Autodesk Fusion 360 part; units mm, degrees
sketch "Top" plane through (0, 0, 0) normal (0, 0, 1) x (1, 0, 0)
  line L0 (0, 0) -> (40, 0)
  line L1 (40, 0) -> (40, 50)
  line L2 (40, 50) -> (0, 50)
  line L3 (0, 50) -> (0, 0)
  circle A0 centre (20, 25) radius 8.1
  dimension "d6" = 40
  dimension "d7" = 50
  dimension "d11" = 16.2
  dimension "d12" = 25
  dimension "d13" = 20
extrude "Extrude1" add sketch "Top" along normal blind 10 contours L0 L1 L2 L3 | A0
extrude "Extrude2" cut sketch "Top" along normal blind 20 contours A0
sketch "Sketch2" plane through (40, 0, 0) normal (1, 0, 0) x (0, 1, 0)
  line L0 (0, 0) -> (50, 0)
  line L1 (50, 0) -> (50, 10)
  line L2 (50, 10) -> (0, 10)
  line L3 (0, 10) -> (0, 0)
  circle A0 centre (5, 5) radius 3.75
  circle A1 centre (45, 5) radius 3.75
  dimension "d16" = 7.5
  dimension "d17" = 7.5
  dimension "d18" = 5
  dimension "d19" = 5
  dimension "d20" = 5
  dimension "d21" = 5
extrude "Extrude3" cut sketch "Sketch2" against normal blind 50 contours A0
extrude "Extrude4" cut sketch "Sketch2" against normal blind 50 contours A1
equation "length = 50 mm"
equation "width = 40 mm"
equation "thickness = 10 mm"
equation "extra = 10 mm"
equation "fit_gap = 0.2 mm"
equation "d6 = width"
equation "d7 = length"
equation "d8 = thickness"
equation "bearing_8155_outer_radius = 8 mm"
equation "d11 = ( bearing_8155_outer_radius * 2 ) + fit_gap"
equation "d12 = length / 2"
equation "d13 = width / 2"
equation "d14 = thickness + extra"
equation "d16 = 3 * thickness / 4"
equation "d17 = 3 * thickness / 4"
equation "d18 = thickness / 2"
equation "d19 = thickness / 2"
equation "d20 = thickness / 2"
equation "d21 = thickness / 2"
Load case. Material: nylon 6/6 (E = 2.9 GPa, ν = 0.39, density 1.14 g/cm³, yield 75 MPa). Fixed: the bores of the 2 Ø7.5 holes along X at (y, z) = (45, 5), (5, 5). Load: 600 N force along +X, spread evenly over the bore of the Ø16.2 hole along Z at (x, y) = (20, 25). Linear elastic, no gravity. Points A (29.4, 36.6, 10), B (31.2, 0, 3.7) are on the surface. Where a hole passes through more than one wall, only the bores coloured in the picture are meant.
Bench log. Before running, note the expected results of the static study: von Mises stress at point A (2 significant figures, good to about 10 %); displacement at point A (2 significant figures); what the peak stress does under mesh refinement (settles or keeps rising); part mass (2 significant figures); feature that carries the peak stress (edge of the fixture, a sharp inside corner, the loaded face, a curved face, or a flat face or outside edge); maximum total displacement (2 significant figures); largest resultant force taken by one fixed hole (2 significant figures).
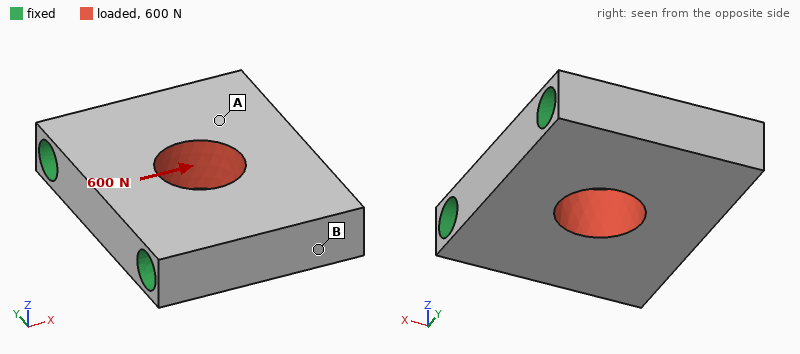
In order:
1.3 MPa
4.2 µm
keeps rising
16 g
edge of the fixture
13 µm
300 N
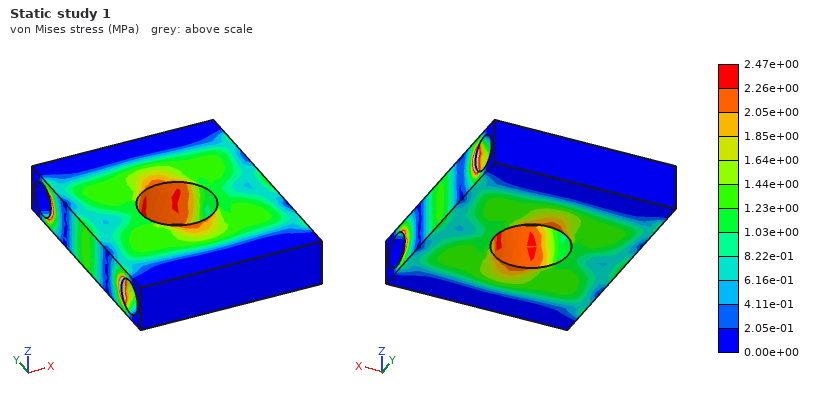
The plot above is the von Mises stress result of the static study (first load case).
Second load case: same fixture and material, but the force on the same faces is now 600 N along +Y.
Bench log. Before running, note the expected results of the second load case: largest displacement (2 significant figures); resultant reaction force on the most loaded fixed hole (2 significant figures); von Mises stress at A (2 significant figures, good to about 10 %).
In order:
5.5 µm
300 N
0.82 MPa
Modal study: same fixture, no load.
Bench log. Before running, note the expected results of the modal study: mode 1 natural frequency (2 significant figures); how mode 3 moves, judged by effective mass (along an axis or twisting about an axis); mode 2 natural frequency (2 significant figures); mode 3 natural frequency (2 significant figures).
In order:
9700 Hz
along X
9800 Hz
14 kHz
